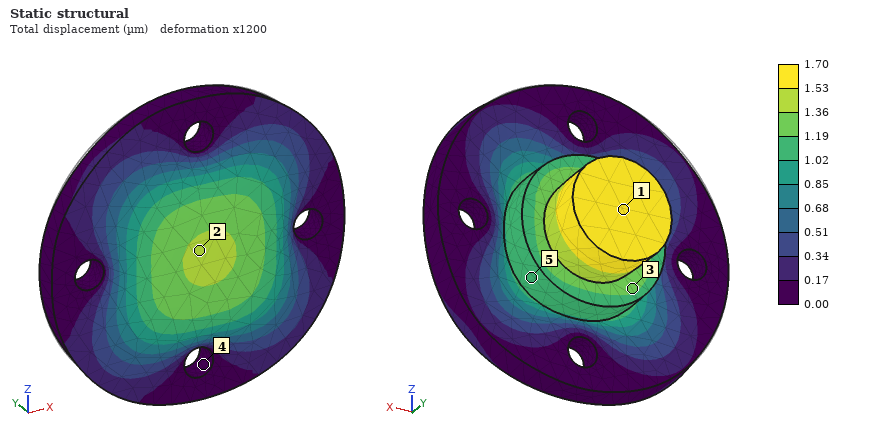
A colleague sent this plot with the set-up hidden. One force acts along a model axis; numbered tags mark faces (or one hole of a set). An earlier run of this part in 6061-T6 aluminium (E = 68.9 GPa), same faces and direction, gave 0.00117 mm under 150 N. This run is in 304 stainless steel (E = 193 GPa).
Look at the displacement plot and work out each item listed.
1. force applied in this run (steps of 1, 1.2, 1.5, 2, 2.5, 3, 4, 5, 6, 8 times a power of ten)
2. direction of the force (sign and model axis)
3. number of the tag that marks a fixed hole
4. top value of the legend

600 N
-Y
4
1.70 µm
